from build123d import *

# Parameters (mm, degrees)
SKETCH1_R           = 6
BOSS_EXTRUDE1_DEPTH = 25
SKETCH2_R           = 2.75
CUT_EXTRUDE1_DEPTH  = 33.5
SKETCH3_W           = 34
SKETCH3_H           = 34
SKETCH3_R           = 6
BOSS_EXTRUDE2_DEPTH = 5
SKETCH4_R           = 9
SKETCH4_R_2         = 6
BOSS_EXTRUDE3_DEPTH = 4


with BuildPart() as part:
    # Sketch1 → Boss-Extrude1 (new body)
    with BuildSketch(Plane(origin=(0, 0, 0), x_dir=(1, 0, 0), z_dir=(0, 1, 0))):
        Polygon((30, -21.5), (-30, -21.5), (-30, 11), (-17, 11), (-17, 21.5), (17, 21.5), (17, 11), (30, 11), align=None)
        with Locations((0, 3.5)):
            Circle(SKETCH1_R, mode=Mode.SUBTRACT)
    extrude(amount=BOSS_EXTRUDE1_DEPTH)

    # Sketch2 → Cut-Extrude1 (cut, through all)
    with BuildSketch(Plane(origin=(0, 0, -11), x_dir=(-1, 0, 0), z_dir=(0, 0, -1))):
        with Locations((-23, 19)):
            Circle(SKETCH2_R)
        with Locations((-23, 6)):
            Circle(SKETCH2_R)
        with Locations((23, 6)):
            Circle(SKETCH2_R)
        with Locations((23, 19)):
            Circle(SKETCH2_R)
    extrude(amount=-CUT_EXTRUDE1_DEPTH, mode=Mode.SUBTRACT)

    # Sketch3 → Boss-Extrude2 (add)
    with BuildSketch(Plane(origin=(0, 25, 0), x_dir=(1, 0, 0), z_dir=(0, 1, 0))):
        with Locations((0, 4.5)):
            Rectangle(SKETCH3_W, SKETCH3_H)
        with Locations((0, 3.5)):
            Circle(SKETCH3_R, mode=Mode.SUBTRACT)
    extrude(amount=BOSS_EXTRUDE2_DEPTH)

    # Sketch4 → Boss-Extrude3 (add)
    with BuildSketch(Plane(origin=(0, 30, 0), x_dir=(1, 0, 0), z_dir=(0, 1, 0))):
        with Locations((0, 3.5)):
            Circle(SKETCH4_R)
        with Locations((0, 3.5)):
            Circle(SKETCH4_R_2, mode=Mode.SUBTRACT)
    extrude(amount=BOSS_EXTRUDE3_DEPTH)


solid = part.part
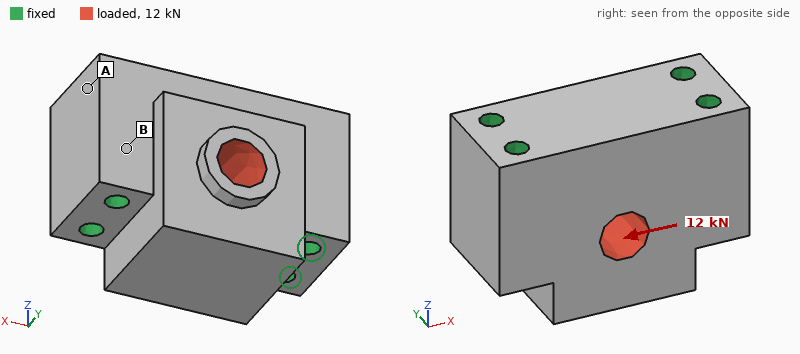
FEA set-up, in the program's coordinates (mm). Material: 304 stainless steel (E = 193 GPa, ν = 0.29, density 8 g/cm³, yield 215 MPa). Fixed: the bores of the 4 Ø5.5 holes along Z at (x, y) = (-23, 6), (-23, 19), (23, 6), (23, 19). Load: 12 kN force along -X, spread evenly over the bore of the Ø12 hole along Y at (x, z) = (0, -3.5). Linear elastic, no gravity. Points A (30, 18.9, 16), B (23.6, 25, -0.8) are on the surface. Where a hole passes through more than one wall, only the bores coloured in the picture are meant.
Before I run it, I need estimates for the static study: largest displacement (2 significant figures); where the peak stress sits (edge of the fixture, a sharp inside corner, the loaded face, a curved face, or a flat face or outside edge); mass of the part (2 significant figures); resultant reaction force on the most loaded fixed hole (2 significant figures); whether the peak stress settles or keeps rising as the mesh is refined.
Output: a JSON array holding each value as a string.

["2.6 µm", "edge of the fixture", "460 g", "3.5 kN", "keeps rising"]
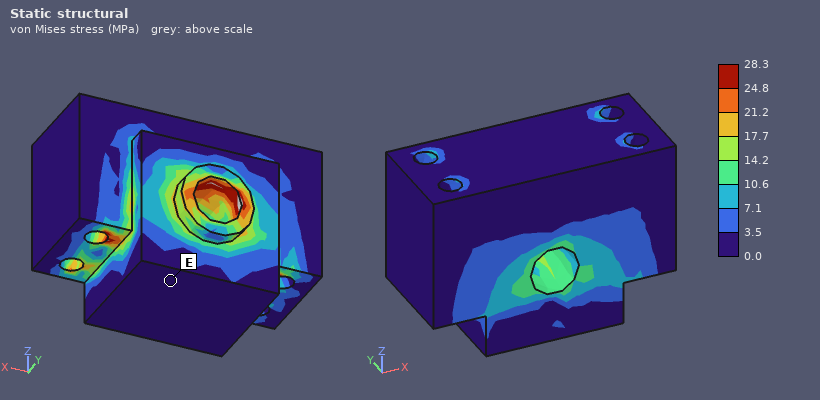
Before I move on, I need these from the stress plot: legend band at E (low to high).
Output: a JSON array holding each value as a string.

["0.0 to 3.5 MPa"]
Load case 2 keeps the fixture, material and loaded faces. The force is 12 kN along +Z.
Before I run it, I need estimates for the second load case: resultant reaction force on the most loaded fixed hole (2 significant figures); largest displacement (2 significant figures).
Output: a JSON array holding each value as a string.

["3.8 kN", "4.3 µm"]
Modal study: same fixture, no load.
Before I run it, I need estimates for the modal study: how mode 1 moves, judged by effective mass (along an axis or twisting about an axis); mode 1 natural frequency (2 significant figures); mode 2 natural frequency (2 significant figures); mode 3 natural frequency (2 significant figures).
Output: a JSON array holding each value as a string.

["along Y", "19 kHz", "28 kHz", "30 kHz"]
